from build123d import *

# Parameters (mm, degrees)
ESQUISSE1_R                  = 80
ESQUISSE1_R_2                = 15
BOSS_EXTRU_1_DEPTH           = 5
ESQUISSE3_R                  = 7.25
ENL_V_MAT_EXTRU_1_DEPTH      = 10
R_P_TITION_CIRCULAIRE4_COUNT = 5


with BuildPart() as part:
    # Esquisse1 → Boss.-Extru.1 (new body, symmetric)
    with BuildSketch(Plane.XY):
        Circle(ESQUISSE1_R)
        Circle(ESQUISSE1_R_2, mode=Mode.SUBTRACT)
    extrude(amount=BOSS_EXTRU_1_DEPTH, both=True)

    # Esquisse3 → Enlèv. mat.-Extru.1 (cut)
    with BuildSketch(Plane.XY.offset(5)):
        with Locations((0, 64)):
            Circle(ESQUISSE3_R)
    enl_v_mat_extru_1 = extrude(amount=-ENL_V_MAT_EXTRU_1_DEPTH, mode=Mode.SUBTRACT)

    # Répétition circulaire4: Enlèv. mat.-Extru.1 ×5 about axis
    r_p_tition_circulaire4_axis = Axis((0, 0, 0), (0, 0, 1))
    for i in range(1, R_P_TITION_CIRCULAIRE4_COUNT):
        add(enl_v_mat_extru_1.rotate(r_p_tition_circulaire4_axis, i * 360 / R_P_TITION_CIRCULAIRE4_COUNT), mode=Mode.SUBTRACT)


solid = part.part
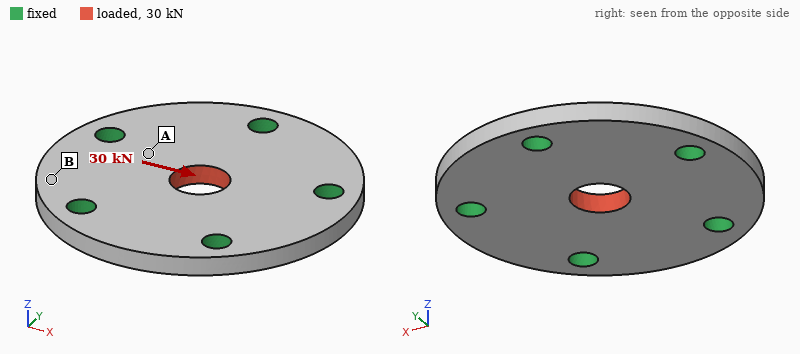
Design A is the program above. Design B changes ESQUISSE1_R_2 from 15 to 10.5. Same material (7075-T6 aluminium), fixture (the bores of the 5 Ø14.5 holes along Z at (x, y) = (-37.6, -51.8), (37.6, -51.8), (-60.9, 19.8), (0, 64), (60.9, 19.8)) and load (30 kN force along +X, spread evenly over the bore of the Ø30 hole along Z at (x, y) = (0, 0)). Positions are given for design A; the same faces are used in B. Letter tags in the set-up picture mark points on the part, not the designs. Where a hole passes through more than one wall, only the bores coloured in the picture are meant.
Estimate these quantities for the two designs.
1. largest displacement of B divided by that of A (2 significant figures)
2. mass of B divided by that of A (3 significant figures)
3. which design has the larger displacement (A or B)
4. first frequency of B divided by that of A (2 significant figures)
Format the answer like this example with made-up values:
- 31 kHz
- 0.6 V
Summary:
- 1.2
- 1.02
- B
- 0.97
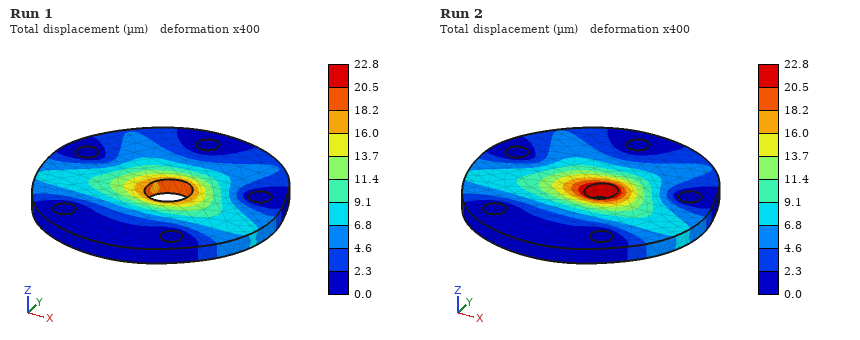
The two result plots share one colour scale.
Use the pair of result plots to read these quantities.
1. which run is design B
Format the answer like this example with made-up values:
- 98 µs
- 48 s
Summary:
- Run 2
